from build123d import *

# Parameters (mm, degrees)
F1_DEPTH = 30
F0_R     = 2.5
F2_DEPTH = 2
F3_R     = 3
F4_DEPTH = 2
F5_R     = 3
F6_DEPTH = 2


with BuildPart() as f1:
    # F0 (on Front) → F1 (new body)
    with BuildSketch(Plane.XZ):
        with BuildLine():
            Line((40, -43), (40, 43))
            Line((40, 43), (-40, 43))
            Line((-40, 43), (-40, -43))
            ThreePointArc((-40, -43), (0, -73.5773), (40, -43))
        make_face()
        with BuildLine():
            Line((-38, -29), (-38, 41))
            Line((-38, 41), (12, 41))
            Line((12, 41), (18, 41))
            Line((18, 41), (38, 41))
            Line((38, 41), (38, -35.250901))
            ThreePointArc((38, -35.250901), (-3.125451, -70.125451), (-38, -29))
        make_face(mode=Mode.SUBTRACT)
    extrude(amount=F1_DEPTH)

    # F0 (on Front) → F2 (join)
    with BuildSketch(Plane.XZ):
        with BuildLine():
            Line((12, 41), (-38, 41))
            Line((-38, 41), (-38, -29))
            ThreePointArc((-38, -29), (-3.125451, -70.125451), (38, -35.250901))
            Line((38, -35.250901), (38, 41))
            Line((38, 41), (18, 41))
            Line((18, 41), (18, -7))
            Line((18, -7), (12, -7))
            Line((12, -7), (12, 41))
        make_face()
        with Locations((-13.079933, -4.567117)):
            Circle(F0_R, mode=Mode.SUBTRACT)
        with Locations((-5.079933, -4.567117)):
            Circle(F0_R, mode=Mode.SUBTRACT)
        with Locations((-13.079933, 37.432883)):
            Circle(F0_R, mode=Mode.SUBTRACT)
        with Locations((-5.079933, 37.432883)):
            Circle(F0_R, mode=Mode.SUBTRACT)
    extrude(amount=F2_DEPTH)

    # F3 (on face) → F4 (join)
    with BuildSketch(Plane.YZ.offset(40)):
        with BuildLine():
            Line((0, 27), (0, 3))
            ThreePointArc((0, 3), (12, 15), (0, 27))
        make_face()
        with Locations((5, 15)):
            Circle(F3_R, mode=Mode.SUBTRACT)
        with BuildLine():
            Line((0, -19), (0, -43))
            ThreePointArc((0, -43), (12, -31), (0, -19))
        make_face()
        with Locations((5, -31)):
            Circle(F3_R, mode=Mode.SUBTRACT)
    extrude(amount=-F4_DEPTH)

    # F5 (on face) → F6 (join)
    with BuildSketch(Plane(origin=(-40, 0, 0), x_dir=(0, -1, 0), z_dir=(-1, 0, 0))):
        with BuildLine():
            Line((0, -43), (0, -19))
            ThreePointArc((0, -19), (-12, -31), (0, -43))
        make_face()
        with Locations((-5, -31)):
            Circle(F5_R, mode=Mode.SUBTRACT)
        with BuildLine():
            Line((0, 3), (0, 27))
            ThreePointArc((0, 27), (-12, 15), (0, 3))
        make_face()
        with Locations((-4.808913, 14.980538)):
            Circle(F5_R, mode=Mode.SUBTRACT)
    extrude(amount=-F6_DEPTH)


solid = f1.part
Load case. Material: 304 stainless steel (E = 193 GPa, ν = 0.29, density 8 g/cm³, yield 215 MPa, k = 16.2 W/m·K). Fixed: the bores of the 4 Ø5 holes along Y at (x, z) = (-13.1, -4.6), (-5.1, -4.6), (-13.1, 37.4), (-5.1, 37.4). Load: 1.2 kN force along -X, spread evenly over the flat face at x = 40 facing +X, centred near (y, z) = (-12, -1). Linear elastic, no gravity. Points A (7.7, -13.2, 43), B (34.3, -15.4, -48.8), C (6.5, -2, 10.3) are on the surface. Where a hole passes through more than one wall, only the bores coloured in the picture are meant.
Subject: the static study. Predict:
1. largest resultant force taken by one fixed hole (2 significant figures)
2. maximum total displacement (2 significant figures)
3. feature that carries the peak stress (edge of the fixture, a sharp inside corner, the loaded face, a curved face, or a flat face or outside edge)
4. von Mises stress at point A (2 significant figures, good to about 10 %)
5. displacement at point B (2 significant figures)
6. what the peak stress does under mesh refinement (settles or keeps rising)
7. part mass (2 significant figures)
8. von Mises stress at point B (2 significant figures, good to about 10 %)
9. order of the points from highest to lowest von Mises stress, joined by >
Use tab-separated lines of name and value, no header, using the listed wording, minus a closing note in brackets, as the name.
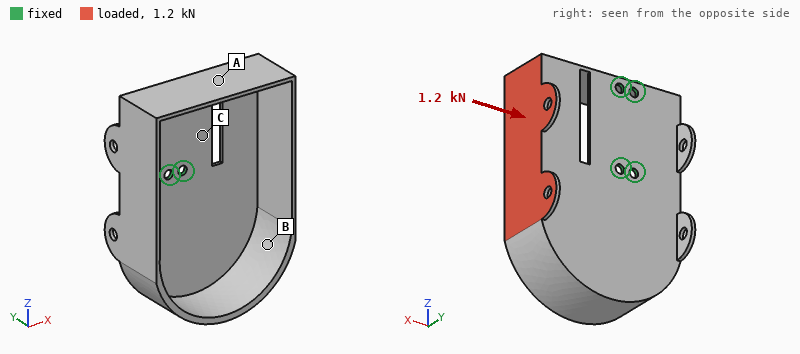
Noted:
largest resultant force taken by one fixed hole	870 N
maximum total displacement	0.54 mm
feature that carries the peak stress	edge of the fixture
von Mises stress at point A	34 MPa
displacement at point B	0.39 mm
what the peak stress does under mesh refinement	keeps rising
part mass	340 g
von Mises stress at point B	66 MPa
order of the points from highest to lowest von Mises stress, joined by >	B > A > C
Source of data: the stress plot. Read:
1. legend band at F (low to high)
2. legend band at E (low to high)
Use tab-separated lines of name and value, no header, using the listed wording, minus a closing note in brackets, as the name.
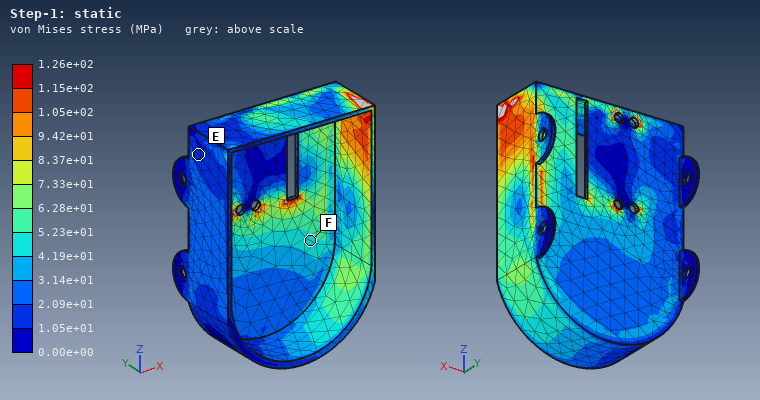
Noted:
legend band at F	4.19e+01 to 5.23e+01 MPa
legend band at E	1.05e+01 to 2.09e+01 MPa
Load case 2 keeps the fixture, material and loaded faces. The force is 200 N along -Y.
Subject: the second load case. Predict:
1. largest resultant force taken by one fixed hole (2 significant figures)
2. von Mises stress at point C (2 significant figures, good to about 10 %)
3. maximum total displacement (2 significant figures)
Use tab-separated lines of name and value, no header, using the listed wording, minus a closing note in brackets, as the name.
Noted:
largest resultant force taken by one fixed hole	680 N
von Mises stress at point C	17 MPa
maximum total displacement	0.34 mm
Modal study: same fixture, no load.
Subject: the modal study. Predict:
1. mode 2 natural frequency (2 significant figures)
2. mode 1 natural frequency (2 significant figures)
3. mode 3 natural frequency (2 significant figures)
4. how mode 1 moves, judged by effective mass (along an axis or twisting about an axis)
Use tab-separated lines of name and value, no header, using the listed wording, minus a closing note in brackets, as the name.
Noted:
mode 2 natural frequency	530 Hz
mode 1 natural frequency	330 Hz
mode 3 natural frequency	1400 Hz
how mode 1 moves, judged by effective mass	along Y
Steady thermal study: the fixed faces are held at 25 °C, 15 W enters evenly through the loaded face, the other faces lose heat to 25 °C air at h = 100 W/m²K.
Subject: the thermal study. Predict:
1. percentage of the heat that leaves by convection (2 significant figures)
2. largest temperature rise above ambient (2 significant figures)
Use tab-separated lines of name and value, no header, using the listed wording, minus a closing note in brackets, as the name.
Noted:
percentage of the heat that leaves by convection	99 %
largest temperature rise above ambient	35 K
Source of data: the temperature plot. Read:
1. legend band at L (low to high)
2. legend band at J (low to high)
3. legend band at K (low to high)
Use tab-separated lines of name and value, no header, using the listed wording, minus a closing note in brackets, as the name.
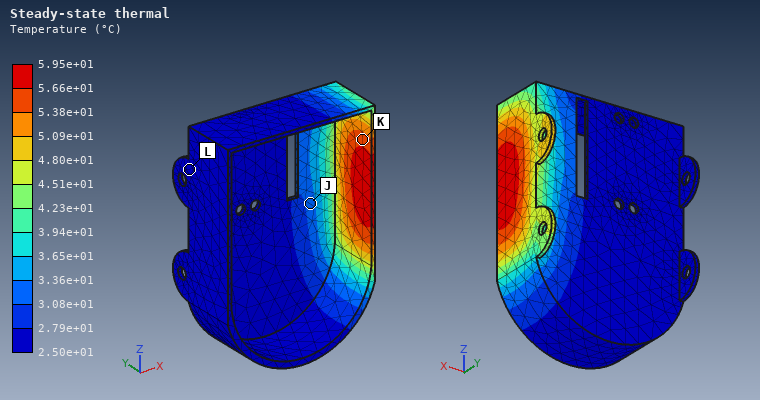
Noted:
legend band at L	2.50e+01 to 2.79e+01 °C
legend band at J	3.08e+01 to 3.36e+01 °C
legend band at K	5.38e+01 to 5.66e+01 °C
